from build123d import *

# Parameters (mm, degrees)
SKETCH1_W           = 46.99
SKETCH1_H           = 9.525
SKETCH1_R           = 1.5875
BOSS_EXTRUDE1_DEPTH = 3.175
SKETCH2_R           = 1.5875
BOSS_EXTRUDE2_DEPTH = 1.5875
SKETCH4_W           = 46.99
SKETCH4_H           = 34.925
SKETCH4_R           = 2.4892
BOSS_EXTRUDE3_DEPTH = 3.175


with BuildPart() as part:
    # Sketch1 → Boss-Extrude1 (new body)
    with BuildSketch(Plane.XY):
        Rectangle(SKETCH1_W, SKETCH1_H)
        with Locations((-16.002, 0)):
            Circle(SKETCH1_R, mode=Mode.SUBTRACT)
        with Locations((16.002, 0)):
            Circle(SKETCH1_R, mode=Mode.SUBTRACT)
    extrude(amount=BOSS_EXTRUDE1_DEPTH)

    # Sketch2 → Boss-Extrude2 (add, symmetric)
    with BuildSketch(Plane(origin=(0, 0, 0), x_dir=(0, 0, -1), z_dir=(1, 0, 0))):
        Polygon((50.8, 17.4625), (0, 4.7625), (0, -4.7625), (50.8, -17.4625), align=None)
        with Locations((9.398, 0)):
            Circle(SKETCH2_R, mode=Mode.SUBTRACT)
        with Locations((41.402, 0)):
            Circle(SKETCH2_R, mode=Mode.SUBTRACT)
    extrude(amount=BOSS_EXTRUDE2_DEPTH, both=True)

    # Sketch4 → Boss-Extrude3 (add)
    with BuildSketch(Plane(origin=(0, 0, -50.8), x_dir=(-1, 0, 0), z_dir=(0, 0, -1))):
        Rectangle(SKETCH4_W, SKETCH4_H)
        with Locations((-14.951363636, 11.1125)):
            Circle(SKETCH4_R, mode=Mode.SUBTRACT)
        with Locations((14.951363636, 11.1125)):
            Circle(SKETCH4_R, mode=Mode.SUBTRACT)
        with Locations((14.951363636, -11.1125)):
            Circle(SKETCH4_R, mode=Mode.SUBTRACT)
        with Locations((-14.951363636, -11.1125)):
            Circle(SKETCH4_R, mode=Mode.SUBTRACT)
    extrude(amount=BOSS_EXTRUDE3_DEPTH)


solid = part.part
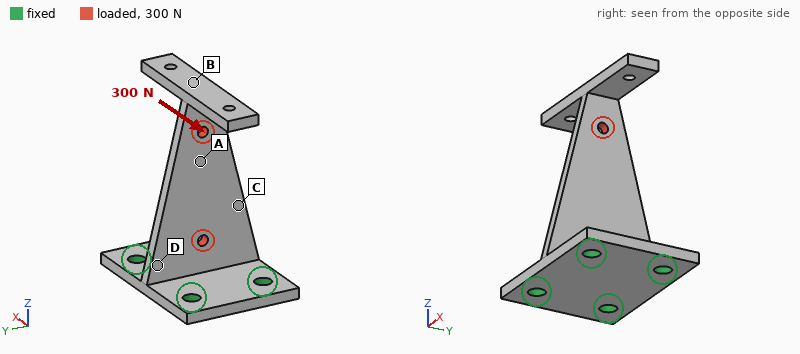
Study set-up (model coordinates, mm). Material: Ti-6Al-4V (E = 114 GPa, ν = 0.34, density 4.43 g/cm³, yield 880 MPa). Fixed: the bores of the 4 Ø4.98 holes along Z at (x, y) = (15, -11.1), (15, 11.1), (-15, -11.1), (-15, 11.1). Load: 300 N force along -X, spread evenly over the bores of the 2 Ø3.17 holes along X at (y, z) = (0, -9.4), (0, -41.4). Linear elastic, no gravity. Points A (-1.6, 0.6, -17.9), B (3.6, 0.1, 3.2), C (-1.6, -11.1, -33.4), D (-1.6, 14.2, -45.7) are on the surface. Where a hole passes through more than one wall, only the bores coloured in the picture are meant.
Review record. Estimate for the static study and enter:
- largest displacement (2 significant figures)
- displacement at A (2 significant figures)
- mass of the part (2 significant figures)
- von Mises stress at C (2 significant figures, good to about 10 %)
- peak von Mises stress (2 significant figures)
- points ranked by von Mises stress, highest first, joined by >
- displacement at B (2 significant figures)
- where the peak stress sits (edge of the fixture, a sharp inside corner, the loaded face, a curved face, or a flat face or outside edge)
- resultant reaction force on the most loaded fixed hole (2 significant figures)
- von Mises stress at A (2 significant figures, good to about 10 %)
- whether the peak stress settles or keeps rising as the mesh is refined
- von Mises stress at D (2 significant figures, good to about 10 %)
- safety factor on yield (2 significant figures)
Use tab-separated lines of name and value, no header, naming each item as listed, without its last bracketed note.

largest displacement	0.85 mm
displacement at A	0.36 mm
mass of the part	44 g
von Mises stress at C	86 MPa
peak von Mises stress	180 MPa
points ranked by von Mises stress, highest first, joined by >	D > C > A > B
displacement at B	0.74 mm
where the peak stress sits	the loaded face
resultant reaction force on the most loaded fixed hole	220 N
von Mises stress at A	47 MPa
whether the peak stress settles or keeps rising as the mesh is refined	settles
von Mises stress at D	110 MPa
safety factor on yield	4.9
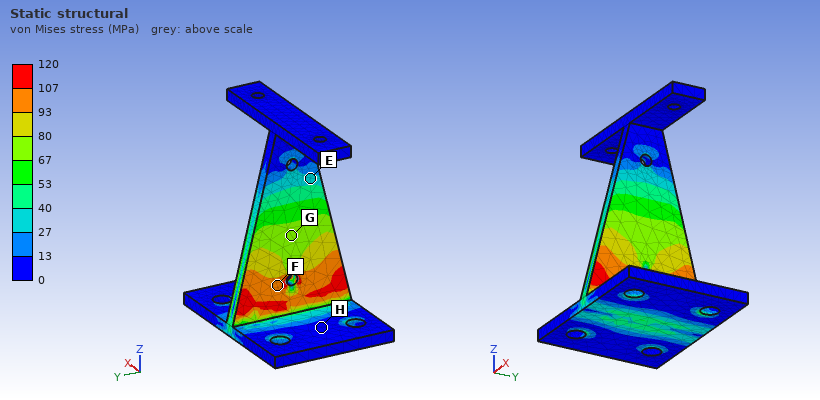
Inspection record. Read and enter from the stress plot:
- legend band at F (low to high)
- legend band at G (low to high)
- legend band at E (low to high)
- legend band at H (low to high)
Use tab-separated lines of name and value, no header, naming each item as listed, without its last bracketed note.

legend band at F	93 to 107 MPa
legend band at G	67 to 80 MPa
legend band at E	27 to 40 MPa
legend band at H	0 to 13 MPa
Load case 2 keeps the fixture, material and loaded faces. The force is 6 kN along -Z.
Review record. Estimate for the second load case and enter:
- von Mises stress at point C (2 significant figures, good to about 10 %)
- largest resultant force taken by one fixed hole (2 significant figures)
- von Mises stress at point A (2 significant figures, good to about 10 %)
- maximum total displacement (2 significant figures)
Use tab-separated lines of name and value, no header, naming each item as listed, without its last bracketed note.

von Mises stress at point C	53 MPa
largest resultant force taken by one fixed hole	1.5 kN
von Mises stress at point A	60 MPa
maximum total displacement	87 µm
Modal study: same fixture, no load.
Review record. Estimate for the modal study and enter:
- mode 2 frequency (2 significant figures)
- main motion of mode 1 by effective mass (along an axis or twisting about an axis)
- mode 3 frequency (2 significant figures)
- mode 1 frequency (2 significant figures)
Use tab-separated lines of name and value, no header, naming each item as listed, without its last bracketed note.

mode 2 frequency	1800 Hz
main motion of mode 1 by effective mass	along X
mode 3 frequency	2200 Hz
mode 1 frequency	650 Hz
